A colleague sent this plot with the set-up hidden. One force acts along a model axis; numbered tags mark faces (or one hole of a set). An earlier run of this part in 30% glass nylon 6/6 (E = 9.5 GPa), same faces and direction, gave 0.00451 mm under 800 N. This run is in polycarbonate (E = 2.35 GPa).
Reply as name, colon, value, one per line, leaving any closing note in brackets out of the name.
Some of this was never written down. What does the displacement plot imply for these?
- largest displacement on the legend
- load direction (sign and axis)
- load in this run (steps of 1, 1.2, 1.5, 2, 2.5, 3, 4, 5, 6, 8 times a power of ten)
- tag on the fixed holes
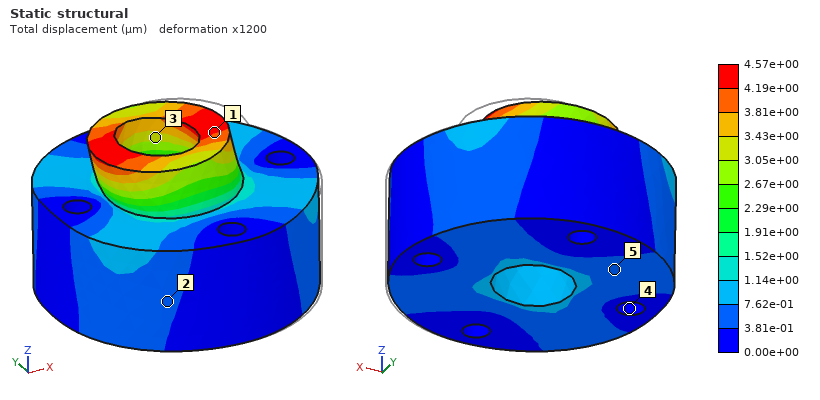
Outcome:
largest displacement on the legend: 4.57e+00 µm
load direction: -X
load in this run: 200 N
tag on the fixed holes: 4
